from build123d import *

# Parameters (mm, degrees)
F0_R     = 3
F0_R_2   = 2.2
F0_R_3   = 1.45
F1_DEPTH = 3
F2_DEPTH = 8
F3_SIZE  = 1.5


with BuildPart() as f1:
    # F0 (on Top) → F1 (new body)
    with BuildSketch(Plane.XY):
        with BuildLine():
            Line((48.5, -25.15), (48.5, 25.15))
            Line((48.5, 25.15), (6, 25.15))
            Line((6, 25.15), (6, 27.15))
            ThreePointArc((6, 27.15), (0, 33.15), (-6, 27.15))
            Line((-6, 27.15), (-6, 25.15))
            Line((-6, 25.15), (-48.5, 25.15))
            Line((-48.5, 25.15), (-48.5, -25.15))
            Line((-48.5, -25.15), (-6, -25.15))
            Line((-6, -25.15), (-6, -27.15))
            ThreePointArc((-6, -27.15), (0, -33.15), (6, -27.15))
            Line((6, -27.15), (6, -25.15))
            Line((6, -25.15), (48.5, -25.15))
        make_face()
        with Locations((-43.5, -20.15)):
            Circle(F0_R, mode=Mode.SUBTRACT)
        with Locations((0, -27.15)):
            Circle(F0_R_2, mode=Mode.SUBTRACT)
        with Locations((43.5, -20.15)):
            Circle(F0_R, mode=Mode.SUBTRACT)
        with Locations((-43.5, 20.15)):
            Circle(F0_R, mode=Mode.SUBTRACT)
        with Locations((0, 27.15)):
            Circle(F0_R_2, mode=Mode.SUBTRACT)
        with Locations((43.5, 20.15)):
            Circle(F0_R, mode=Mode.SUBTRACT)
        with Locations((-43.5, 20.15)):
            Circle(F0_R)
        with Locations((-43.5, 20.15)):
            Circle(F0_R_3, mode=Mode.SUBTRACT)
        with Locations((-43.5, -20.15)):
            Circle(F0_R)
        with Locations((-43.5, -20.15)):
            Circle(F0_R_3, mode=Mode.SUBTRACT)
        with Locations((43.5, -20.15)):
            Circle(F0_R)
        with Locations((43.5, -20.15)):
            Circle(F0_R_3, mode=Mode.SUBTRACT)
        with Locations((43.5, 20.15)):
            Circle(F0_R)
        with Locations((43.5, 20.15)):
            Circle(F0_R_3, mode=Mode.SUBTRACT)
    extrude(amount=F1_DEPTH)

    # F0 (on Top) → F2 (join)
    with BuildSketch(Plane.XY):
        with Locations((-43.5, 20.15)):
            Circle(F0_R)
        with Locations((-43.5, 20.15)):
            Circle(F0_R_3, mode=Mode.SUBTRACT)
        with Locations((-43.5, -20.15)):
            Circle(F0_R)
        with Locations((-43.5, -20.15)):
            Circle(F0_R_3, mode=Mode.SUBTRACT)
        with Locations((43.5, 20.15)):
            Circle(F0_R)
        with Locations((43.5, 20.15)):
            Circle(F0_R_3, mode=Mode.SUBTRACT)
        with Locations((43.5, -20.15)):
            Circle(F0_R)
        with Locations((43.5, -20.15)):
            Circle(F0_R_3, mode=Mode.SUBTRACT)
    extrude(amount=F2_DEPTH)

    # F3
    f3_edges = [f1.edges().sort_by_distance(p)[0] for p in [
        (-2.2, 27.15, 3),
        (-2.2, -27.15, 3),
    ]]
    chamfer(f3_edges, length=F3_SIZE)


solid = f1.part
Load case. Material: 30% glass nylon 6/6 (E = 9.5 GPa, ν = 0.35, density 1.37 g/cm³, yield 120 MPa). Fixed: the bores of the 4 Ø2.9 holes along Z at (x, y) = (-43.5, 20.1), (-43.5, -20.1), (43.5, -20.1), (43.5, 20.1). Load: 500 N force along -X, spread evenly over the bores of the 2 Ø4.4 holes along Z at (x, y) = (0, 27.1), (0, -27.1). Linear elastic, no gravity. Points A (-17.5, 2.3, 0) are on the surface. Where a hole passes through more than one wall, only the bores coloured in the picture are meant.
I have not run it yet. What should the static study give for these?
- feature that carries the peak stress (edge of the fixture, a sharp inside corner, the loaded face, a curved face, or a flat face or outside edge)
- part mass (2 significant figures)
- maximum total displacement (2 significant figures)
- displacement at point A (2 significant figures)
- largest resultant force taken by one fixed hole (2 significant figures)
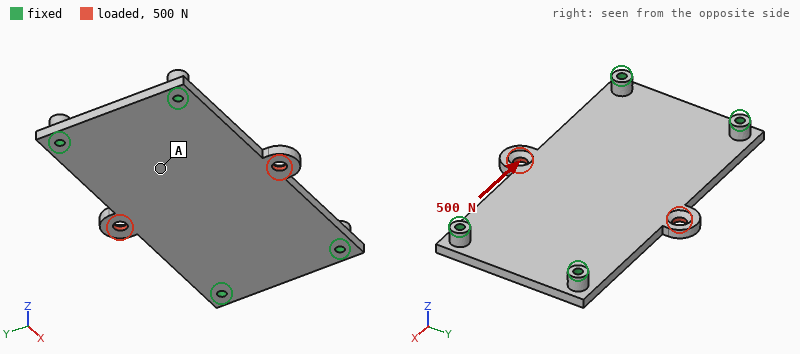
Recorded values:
the loaded face
21 g
50 µm
9.9 µm
130 N
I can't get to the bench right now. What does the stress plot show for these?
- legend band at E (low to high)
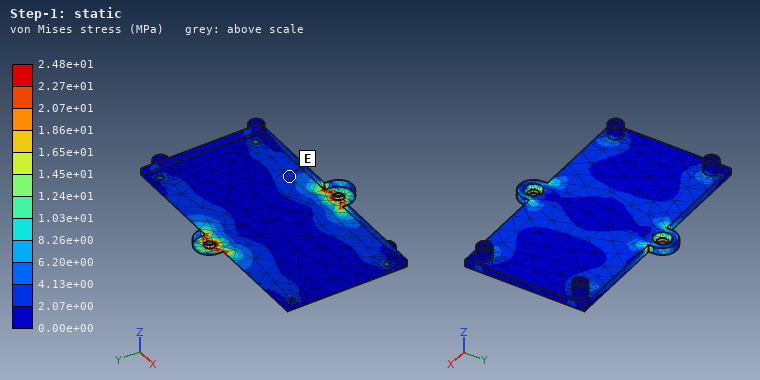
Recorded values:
2.07e+00 to 4.13e+00 MPa
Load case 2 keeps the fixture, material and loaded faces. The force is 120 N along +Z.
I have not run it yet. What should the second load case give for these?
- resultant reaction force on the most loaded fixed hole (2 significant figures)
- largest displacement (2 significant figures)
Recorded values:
32 N
0.76 mm
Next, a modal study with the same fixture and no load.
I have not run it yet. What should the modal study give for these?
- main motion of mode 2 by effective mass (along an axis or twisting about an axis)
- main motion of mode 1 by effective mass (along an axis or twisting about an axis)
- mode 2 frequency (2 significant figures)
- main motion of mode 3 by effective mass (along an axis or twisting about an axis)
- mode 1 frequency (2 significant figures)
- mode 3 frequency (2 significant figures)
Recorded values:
twisting about X
along Z
1500 Hz
twisting about Y
960 Hz
2700 Hz
